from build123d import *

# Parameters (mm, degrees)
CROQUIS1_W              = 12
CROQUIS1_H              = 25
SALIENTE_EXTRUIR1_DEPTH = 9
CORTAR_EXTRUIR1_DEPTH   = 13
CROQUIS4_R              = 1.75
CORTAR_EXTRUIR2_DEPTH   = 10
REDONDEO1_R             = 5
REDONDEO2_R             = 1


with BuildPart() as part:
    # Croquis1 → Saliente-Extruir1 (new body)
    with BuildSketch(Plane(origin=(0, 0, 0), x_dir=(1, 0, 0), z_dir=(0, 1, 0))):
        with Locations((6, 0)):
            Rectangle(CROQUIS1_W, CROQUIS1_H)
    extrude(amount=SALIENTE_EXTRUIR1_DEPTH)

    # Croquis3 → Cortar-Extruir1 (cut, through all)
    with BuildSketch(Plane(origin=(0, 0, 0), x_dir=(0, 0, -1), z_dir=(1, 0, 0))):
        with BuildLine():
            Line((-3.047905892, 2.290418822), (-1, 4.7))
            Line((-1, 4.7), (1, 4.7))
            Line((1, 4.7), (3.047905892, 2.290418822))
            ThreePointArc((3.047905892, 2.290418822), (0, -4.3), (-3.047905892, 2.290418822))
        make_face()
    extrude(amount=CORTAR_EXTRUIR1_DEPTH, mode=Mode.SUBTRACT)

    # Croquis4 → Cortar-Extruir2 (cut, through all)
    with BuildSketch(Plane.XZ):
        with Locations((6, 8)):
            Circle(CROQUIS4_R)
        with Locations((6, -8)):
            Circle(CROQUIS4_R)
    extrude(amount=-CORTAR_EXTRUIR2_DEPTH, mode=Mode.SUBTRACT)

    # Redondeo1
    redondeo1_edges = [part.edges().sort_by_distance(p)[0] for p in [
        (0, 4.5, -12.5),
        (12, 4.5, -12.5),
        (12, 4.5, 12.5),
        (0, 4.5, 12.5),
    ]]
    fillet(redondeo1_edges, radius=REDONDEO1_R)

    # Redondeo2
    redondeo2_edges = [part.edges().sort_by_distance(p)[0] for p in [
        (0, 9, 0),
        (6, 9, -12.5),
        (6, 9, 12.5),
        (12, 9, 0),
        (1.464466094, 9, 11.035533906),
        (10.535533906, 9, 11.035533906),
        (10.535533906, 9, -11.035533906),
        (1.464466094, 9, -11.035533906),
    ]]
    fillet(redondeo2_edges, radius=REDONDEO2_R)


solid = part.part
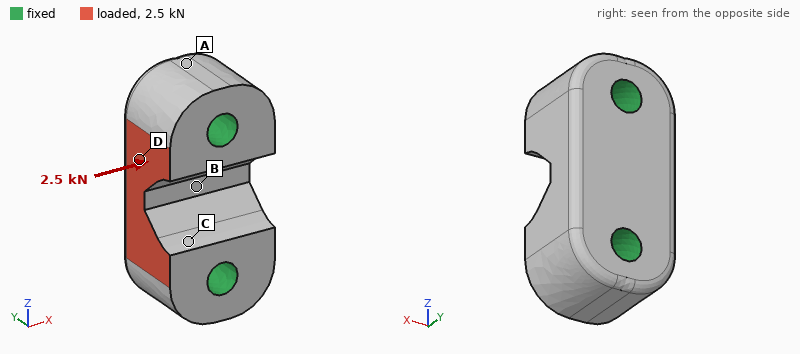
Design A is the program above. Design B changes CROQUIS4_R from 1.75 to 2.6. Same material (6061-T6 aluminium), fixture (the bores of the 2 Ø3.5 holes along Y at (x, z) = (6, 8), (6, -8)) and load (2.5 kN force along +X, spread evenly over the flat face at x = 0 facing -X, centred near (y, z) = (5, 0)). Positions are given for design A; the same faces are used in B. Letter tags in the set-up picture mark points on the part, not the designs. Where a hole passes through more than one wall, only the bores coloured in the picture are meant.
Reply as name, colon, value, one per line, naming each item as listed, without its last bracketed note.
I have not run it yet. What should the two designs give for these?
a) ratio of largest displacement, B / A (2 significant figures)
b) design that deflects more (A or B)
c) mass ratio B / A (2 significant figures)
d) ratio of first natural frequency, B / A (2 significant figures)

ratio of largest displacement, B / A: 0.78
design that deflects more: A
mass ratio B / A: 0.90
ratio of first natural frequency, B / A: 1.3
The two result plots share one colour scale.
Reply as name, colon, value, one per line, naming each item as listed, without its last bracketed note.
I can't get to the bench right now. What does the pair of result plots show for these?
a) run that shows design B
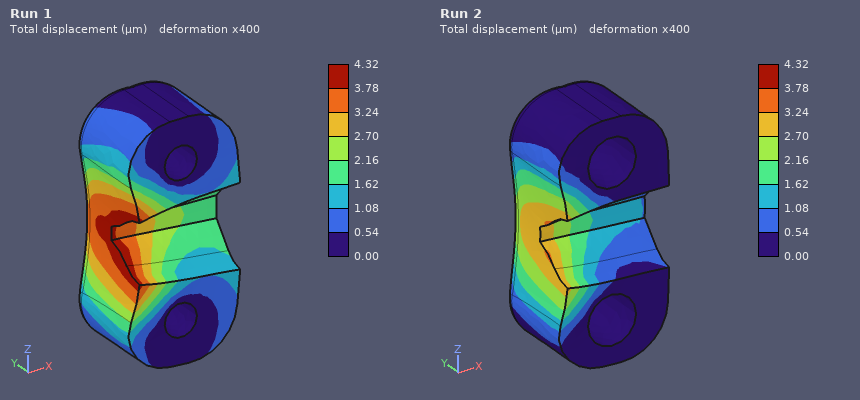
run that shows design B: Run 2
